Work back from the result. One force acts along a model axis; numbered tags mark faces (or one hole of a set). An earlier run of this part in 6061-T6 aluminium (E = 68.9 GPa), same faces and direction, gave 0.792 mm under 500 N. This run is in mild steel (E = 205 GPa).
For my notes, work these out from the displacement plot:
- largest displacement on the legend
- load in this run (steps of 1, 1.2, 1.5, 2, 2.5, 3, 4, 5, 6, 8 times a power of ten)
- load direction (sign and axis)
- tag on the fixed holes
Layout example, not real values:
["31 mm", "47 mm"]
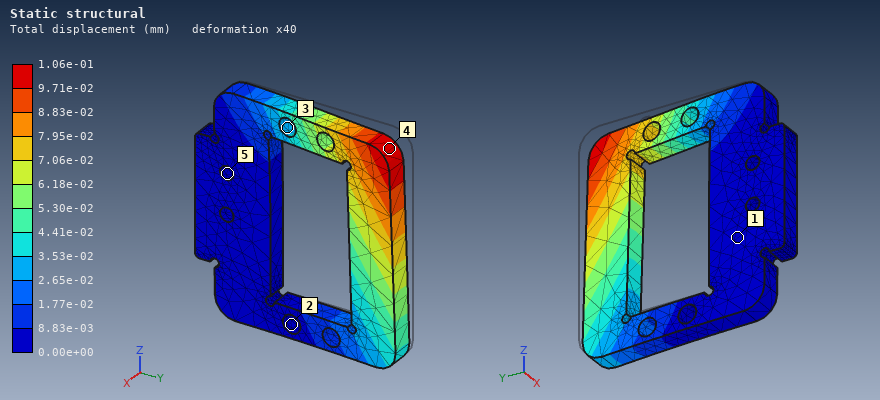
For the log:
["1.06e-01 mm", "200 N", "+X", "5"]
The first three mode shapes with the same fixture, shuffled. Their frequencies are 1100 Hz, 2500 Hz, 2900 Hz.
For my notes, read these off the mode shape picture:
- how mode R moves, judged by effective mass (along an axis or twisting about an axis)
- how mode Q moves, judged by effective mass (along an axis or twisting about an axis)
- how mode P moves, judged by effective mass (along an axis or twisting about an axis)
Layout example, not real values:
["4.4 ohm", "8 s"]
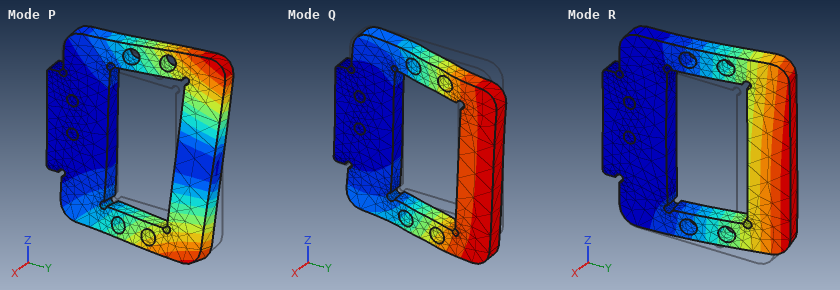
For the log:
["along X", "along Z", "twisting about Y"]
